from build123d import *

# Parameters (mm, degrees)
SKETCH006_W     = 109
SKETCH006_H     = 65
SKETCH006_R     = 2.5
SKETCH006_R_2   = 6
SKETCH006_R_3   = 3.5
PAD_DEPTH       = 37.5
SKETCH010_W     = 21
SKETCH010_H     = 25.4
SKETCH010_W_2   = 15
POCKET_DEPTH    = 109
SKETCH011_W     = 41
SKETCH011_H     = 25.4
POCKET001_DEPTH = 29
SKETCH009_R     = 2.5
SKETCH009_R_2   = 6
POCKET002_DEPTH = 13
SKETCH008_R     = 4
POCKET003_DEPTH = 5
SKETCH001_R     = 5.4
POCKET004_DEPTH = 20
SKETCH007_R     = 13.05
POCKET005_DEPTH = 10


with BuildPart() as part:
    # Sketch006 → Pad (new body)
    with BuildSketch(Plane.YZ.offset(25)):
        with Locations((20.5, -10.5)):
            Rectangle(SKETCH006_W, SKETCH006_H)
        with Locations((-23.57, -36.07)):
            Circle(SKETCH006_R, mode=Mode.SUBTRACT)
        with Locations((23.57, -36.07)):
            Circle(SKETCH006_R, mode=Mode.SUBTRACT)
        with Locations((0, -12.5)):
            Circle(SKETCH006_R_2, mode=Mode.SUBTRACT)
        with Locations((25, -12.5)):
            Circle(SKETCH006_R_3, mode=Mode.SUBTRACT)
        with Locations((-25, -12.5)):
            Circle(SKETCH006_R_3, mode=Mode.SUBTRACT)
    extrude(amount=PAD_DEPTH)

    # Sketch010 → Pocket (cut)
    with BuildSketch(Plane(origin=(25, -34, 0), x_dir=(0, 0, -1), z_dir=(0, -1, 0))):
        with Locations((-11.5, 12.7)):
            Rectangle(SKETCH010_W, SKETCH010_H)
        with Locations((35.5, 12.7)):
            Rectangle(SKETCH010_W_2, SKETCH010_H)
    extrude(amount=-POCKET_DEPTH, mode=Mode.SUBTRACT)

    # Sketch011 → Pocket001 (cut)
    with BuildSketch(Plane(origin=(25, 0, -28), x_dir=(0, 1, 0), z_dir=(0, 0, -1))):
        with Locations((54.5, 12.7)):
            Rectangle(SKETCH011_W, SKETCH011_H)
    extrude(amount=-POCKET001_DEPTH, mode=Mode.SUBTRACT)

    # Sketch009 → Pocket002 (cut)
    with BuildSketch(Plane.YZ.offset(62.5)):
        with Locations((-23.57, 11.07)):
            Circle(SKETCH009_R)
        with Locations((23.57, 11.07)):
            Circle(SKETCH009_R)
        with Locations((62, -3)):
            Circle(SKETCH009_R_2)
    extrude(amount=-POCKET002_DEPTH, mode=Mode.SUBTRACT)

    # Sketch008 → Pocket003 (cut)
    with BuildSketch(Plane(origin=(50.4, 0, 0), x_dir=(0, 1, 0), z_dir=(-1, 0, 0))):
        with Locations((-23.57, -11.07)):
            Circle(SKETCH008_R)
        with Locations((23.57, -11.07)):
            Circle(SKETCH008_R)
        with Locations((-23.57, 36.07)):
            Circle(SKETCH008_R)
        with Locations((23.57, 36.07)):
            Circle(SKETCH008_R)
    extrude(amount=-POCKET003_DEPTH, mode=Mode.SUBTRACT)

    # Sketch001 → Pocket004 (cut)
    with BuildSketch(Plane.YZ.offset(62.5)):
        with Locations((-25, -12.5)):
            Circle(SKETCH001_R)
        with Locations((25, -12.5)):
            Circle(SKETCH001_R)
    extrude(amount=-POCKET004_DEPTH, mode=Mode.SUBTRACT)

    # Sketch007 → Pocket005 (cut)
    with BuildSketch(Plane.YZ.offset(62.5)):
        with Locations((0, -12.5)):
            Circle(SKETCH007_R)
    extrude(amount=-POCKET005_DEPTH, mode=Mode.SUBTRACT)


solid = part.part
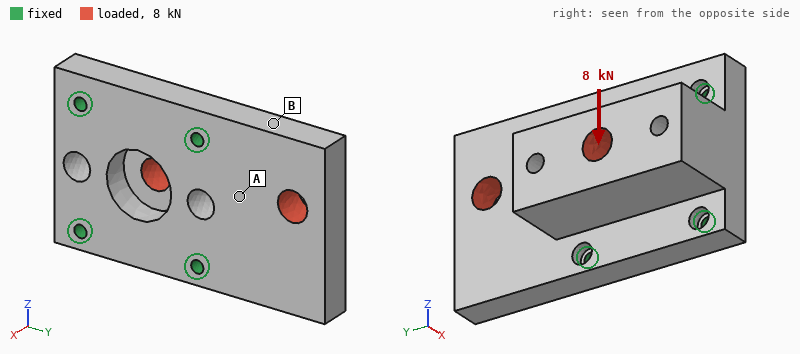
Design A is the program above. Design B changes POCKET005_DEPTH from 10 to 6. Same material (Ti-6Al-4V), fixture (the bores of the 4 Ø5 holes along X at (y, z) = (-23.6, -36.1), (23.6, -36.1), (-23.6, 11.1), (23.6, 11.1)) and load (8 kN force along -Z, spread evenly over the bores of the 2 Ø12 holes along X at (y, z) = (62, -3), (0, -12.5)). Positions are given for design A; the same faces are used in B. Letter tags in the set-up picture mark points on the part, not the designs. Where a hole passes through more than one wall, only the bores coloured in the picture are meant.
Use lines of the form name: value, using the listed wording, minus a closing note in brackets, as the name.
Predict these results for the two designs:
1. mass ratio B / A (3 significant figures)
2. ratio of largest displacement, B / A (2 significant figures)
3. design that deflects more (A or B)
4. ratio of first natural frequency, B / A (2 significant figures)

mass ratio B / A: 1.01
ratio of largest displacement, B / A: 0.91
design that deflects more: A
ratio of first natural frequency, B / A: 1.0
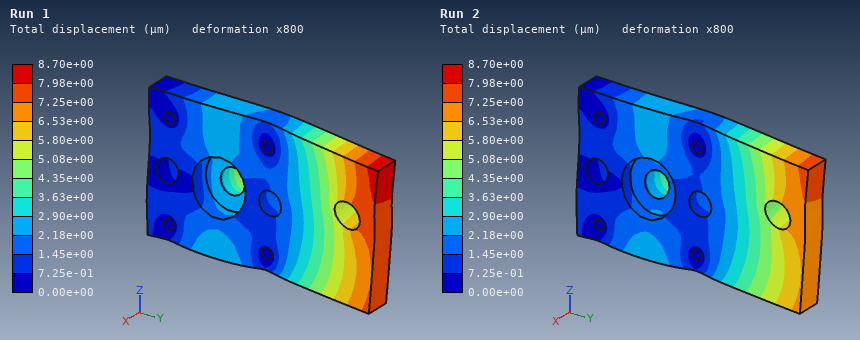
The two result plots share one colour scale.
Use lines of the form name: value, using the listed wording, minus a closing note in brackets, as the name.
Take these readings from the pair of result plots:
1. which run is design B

which run is design B: Run 2
